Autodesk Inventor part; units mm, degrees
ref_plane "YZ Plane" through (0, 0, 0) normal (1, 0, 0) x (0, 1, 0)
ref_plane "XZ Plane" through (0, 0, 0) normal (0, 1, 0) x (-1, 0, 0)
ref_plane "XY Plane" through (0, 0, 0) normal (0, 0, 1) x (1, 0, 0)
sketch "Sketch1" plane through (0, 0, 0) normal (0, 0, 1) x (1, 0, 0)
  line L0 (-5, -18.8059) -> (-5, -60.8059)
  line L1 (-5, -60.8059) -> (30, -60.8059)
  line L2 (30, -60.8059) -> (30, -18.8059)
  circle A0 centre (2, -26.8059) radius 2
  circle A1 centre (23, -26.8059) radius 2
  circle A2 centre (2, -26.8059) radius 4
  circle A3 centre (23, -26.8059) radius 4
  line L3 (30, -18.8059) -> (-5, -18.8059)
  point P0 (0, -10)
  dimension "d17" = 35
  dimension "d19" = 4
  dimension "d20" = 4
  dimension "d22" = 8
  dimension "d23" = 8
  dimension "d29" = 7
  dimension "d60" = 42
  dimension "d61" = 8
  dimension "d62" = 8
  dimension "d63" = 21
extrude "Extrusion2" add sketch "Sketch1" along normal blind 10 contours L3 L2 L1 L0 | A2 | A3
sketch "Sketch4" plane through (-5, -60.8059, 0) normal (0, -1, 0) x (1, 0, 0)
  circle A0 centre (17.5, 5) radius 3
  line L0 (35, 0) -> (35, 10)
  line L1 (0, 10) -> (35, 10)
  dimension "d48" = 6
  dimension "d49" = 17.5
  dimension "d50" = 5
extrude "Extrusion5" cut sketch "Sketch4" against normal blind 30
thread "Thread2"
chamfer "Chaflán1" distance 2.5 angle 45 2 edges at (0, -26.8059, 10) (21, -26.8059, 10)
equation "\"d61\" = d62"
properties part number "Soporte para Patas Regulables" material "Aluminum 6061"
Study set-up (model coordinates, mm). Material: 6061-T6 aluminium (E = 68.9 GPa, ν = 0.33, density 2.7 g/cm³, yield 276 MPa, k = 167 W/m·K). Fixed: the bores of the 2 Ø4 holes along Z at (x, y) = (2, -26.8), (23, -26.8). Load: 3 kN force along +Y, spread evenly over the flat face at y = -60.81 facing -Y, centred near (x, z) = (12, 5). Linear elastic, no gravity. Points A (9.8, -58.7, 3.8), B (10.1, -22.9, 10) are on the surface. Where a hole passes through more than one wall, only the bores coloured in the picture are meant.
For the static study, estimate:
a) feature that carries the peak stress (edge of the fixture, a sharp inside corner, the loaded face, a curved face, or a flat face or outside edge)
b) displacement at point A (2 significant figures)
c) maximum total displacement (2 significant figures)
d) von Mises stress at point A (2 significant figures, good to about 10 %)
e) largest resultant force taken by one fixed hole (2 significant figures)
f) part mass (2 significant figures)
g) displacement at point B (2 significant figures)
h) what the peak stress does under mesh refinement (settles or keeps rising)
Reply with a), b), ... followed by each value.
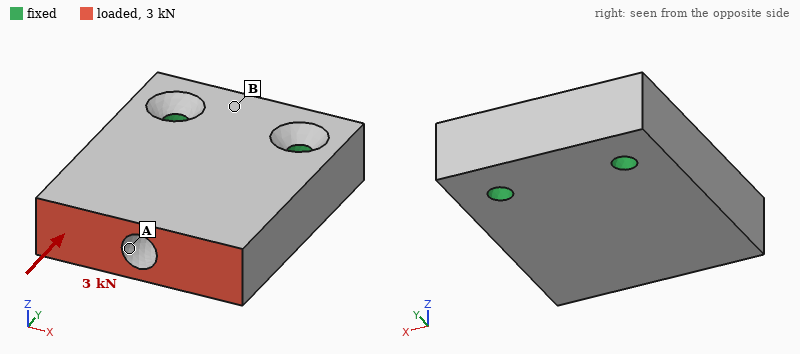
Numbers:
a) edge of the fixture
b) 5.9 µm
c) 7.1 µm
d) 9.3 MPa
e) 1.5 kN
f) 36 g
g) 1.5 µm
h) keeps rising
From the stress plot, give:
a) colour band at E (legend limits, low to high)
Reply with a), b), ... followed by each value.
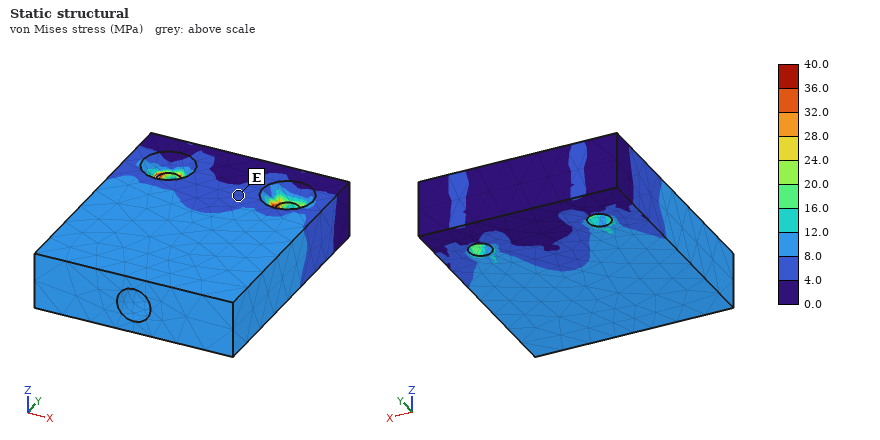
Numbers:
a) 4.0 to 8.0 MPa
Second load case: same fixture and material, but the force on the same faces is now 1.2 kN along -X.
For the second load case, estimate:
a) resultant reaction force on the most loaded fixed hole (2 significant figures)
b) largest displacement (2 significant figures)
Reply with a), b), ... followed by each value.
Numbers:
a) 1.8 kN
b) 19 µm
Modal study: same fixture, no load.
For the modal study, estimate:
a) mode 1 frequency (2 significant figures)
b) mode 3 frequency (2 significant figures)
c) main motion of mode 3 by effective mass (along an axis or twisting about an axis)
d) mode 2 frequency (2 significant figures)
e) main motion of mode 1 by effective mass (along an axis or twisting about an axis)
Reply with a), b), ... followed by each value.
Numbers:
a) 5700 Hz
b) 14 kHz
c) along X
d) 12 kHz
e) along Z
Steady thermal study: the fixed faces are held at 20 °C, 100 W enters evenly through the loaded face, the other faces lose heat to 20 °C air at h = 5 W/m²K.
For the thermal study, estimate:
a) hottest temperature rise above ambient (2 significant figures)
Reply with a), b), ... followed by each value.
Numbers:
a) 65 K
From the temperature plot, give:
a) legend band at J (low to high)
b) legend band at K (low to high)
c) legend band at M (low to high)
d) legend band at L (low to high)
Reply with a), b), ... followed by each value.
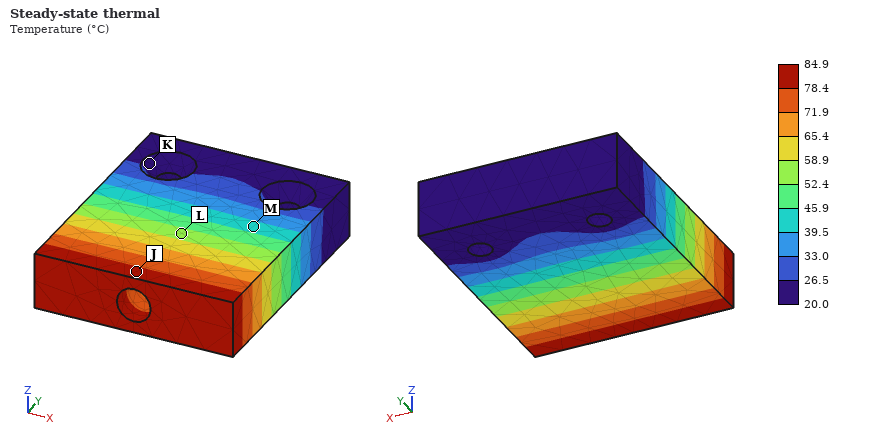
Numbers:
a) 78.4 to 84.9 °C
b) 20.0 to 26.5 °C
c) 39.5 to 45.9 °C
d) 52.4 to 58.9 °C
